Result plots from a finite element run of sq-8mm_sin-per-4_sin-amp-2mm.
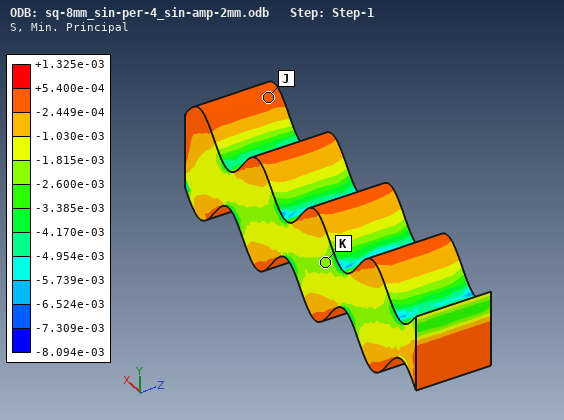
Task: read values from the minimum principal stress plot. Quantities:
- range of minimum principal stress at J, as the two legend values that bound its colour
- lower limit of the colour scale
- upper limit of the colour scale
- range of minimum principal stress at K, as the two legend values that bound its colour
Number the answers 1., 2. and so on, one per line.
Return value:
1. -2.449e-04 to +5.400e-04
2. -8.094e-03
3. +1.325e-03
4. -2.600e-03 to -1.815e-03
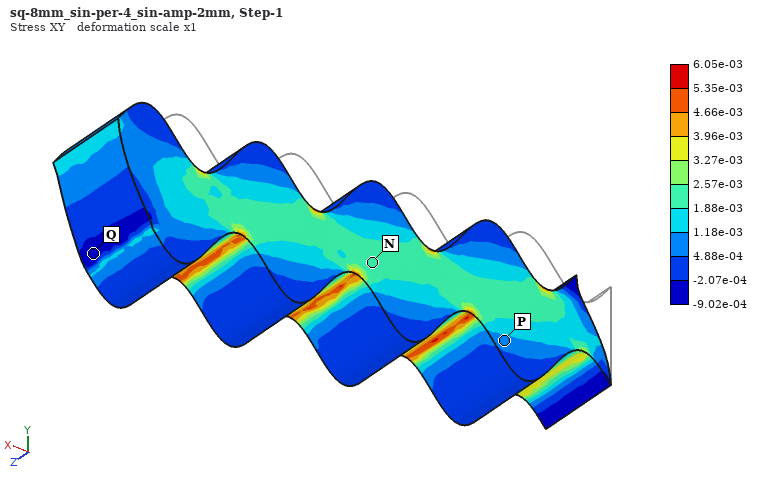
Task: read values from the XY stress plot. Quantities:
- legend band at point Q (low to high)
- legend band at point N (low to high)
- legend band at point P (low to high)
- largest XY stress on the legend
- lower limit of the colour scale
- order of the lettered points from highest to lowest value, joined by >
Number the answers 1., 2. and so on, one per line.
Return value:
1. -9.02e-04 to -2.07e-04
2. 1.88e-03 to 2.57e-03
3. 4.88e-04 to 1.18e-03
4. 6.05e-03
5. -9.02e-04
6. N > P > Q
